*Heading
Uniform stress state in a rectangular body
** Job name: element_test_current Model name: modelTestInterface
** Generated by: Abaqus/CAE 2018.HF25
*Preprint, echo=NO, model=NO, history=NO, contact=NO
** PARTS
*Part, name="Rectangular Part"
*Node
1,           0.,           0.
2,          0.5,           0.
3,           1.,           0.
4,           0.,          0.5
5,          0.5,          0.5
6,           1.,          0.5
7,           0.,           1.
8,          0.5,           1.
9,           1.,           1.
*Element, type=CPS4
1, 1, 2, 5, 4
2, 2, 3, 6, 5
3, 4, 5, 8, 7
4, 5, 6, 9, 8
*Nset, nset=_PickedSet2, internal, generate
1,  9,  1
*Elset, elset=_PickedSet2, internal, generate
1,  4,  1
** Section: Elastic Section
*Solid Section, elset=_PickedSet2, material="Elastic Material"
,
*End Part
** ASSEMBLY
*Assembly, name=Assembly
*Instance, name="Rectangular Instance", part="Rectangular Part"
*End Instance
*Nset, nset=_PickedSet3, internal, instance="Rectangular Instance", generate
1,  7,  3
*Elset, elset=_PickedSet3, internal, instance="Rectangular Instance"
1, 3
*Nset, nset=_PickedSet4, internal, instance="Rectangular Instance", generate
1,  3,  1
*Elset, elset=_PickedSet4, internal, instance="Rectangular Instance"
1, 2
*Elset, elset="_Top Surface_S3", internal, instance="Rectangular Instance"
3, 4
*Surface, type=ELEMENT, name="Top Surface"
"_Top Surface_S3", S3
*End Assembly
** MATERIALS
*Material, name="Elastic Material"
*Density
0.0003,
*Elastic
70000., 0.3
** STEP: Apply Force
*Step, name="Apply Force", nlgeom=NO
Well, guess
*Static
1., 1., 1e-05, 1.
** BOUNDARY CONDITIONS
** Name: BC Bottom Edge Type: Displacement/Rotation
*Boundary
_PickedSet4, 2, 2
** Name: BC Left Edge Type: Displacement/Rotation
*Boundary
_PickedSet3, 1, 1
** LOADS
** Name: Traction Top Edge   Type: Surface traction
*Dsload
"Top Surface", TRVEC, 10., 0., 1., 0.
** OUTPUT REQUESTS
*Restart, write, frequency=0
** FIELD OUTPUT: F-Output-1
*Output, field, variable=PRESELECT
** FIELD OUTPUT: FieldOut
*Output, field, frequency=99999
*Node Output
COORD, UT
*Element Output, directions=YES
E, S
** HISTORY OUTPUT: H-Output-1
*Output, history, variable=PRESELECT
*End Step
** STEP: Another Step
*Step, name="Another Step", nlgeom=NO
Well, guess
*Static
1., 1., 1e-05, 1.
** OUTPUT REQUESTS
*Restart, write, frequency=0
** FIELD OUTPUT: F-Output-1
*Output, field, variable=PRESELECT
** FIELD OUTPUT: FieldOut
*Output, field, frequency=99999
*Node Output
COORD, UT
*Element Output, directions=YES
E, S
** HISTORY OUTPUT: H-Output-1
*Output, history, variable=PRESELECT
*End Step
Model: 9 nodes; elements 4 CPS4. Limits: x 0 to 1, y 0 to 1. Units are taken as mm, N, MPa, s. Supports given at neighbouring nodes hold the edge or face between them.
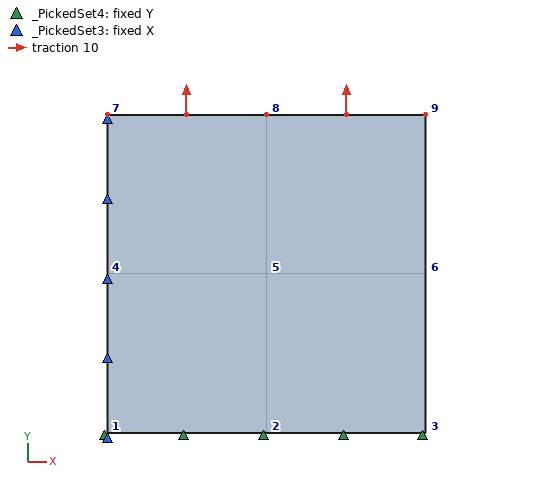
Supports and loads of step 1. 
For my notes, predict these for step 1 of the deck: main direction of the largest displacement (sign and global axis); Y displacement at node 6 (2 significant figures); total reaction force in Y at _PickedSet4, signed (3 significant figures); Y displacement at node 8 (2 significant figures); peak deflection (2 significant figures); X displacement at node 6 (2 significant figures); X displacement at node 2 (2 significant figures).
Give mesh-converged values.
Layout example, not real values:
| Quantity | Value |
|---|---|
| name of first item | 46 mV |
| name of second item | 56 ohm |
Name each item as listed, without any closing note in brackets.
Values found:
| Quantity | Value |
|---|---|
| main direction of the largest displacement | +Y |
| Y displacement at node 6 | 7.1e-05 mm |
| total reaction force in Y at _PickedSet4, signed | -10.0 N |
| Y displacement at node 8 | 1.4e-04 mm |
| peak deflection | 1.5e-04 mm |
| X displacement at node 6 | -4.3e-05 mm |
| X displacement at node 2 | -2.1e-05 mm |
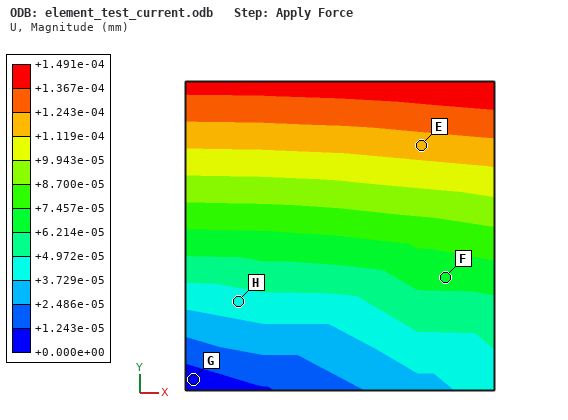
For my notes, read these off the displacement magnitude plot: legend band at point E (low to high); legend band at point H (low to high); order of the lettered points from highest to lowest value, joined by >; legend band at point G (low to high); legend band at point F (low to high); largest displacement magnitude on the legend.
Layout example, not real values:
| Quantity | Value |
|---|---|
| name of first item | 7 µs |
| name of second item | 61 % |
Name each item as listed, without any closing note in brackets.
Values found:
| Quantity | Value |
|---|---|
| legend band at point E | +1.119e-04 to +1.243e-04 mm |
| legend band at point H | +3.729e-05 to +4.972e-05 mm |
| order of the lettered points from highest to lowest value, joined by > | E > F > H > G |
| legend band at point G | +0.000e+00 to +1.243e-05 mm |
| legend band at point F | +6.214e-05 to +7.457e-05 mm |
| largest displacement magnitude on the legend | +1.491e-04 mm |
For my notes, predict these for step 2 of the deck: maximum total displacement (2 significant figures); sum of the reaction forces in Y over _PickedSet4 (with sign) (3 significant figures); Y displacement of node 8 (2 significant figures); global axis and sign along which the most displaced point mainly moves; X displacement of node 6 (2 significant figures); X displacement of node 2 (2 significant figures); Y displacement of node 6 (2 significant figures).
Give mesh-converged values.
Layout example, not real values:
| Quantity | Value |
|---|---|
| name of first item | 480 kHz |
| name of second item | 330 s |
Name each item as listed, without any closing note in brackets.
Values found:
| Quantity | Value |
|---|---|
| maximum total displacement | 1.5e-04 mm |
| sum of the reaction forces in Y over _PickedSet4 (with sign) | -10.0 N |
| Y displacement of node 8 | 1.4e-04 mm |
| global axis and sign along which the most displaced point mainly moves | +Y |
| X displacement of node 6 | -4.3e-05 mm |
| X displacement of node 2 | -2.1e-05 mm |
| Y displacement of node 6 | 7.1e-05 mm |
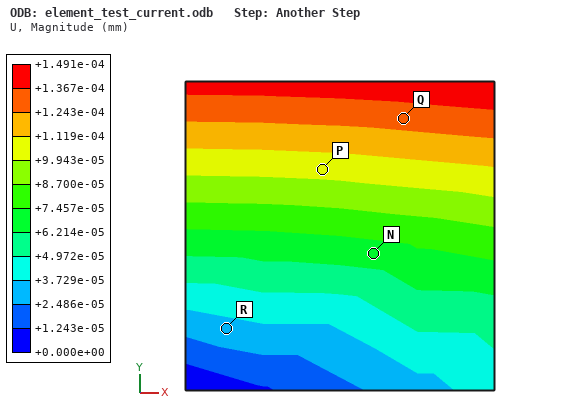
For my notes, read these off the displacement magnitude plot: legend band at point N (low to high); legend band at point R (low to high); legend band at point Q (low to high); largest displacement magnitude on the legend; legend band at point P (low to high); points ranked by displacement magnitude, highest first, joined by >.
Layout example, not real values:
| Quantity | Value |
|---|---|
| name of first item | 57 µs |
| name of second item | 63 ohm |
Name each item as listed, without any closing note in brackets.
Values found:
| Quantity | Value |
|---|---|
| legend band at point N | +6.214e-05 to +7.457e-05 mm |
| legend band at point R | +2.486e-05 to +3.729e-05 mm |
| legend band at point Q | +1.243e-04 to +1.367e-04 mm |
| largest displacement magnitude on the legend | +1.491e-04 mm |
| legend band at point P | +9.943e-05 to +1.119e-04 mm |
| points ranked by displacement magnitude, highest first, joined by > | Q > P > N > R |
